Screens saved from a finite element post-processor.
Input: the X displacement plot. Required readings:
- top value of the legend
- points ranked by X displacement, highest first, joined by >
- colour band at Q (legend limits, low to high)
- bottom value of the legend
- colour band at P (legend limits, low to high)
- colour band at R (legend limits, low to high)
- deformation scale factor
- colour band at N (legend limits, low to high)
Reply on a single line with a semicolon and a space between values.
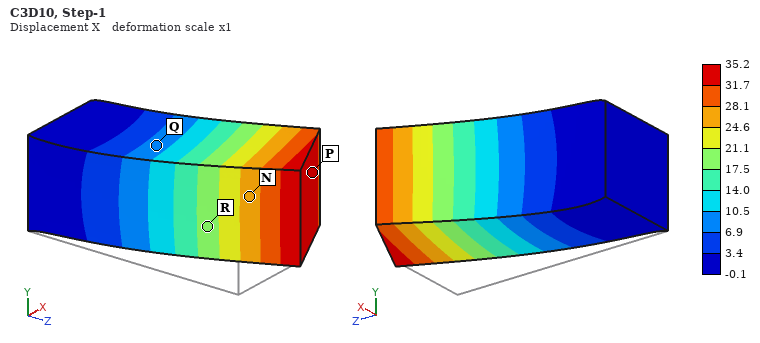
35.2; P > N > R > Q; 6.9 to 10.5; -0.1; 31.7 to 35.2; 17.5 to 21.1; 1; 24.6 to 28.1
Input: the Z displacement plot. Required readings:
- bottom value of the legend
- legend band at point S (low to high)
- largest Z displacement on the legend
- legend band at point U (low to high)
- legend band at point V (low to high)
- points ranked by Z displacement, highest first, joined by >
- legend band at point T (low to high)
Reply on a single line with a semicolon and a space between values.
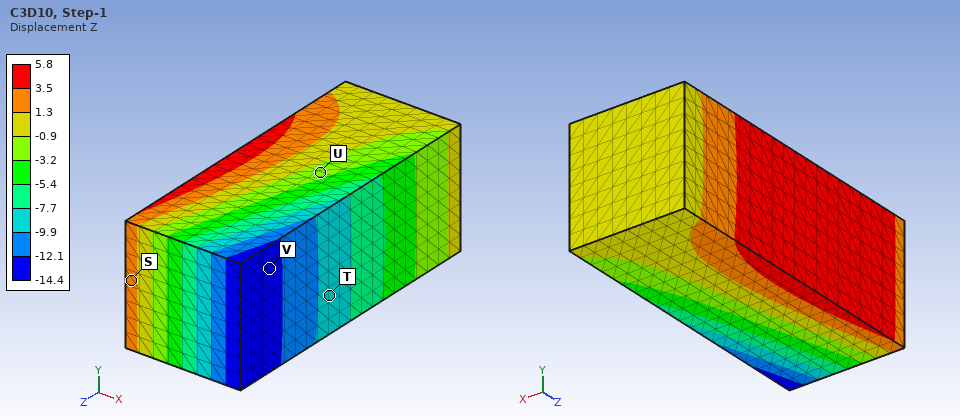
-14.4; 1.3 to 3.5; 5.8; -3.2 to -0.9; -14.4 to -12.1; S > U > T > V; -9.9 to -7.7
